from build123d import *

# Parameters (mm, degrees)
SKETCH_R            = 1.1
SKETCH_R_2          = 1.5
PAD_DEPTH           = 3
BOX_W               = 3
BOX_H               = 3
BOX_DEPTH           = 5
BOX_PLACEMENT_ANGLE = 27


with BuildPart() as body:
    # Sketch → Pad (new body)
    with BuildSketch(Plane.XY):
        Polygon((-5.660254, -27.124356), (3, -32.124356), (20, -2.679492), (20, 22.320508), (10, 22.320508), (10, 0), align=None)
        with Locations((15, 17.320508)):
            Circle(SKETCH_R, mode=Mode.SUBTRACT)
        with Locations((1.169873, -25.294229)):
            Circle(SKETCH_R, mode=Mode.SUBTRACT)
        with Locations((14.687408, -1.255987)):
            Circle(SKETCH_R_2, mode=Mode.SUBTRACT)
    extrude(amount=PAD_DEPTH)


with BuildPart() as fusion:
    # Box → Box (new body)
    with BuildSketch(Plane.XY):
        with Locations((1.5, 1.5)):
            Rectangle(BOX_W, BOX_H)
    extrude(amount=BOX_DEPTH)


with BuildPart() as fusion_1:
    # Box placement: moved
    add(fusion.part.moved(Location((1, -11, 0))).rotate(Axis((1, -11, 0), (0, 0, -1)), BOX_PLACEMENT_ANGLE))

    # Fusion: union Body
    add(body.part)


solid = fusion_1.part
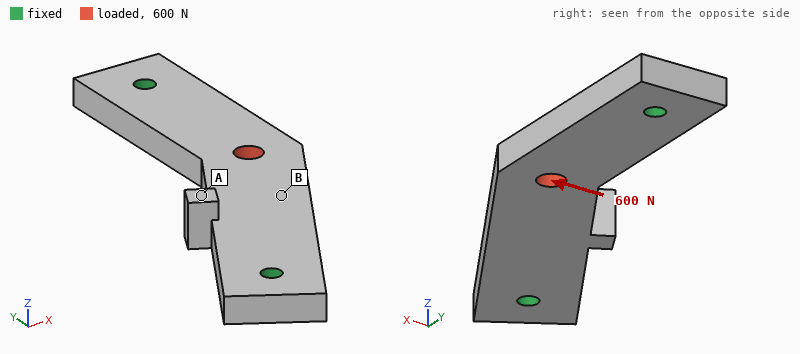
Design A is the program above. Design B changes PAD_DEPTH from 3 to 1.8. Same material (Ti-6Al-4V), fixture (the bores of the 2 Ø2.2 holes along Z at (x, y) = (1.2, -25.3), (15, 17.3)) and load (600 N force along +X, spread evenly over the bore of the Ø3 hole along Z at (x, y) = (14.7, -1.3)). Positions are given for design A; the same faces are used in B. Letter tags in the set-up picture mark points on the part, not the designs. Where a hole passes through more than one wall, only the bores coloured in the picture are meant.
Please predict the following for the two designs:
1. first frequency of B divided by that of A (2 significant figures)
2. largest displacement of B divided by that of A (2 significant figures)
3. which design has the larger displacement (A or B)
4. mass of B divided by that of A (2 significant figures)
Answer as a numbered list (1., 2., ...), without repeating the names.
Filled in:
1. 0.62
2. 1.7
3. B
4. 0.61
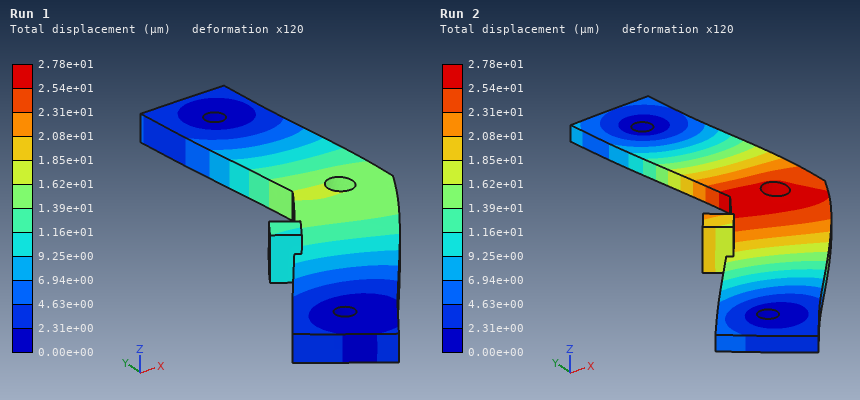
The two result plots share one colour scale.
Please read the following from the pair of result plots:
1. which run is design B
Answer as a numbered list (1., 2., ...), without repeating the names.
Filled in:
1. Run 2
